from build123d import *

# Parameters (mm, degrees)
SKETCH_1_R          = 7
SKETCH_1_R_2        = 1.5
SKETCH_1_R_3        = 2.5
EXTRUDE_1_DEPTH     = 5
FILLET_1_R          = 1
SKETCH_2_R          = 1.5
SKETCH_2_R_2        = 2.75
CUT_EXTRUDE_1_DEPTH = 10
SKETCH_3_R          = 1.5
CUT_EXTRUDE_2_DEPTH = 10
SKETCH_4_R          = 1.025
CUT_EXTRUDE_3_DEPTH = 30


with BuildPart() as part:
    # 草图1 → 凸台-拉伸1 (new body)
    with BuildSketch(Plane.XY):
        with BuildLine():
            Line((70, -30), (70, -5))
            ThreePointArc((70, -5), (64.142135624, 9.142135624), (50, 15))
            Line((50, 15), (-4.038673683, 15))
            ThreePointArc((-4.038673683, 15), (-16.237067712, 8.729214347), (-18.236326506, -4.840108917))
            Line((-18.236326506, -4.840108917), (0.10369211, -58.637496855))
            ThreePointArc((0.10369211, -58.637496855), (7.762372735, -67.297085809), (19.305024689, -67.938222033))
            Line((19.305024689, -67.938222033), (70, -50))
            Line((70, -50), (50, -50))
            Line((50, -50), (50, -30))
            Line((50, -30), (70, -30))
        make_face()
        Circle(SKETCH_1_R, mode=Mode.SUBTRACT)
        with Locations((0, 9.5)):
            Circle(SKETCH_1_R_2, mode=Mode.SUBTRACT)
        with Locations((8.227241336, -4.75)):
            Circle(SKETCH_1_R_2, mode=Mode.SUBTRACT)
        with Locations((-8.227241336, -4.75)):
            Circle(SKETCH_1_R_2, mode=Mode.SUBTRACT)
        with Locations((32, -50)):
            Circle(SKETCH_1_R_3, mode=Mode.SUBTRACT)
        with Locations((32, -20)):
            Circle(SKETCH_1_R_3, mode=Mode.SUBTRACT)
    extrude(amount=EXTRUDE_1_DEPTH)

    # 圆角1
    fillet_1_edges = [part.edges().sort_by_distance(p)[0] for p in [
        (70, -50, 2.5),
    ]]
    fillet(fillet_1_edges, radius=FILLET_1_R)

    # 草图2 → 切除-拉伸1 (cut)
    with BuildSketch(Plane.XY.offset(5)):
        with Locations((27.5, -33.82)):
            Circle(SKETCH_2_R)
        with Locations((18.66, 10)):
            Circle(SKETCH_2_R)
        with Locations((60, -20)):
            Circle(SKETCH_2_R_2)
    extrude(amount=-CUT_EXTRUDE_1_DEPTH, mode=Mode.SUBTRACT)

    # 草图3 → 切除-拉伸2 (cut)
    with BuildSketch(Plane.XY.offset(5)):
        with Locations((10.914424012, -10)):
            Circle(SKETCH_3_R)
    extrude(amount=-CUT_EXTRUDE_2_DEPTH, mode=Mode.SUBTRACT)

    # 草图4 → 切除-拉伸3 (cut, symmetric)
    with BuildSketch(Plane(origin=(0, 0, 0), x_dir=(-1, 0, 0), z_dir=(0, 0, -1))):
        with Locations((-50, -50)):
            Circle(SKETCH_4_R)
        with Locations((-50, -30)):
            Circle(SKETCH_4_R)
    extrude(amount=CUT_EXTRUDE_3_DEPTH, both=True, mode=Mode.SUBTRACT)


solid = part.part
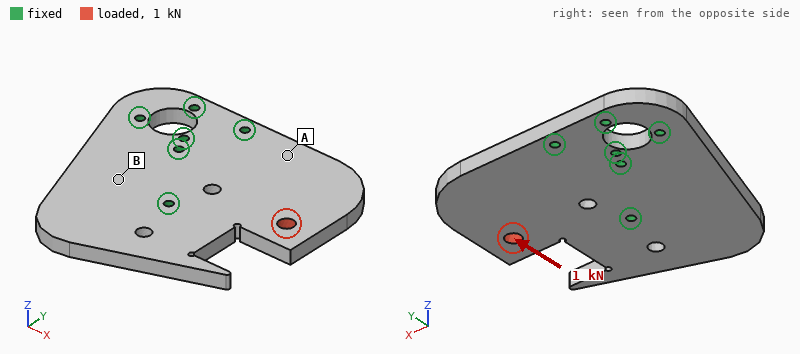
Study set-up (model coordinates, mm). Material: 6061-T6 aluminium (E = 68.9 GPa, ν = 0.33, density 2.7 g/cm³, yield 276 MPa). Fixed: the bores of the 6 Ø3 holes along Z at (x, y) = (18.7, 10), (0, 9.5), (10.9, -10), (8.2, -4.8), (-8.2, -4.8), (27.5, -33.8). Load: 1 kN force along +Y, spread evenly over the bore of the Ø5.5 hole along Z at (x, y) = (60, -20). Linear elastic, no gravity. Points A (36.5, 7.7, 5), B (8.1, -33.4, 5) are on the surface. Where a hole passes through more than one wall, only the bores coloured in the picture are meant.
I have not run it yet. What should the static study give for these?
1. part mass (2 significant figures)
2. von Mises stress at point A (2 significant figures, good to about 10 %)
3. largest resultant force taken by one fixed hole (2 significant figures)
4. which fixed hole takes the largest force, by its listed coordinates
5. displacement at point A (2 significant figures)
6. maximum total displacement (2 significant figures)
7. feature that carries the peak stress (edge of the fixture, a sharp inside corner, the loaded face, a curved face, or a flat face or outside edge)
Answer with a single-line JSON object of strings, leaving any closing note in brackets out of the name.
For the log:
{"part mass": "73 g", "von Mises stress at point A": "7.3 MPa", "largest resultant force taken by one fixed hole": "1.1 kN", "which fixed hole takes the largest force, by its listed coordinates": "(27.5, -33.8)", "displacement at point A": "4.0 µm", "maximum total displacement": "14 µm", "feature that carries the peak stress": "a curved face"}
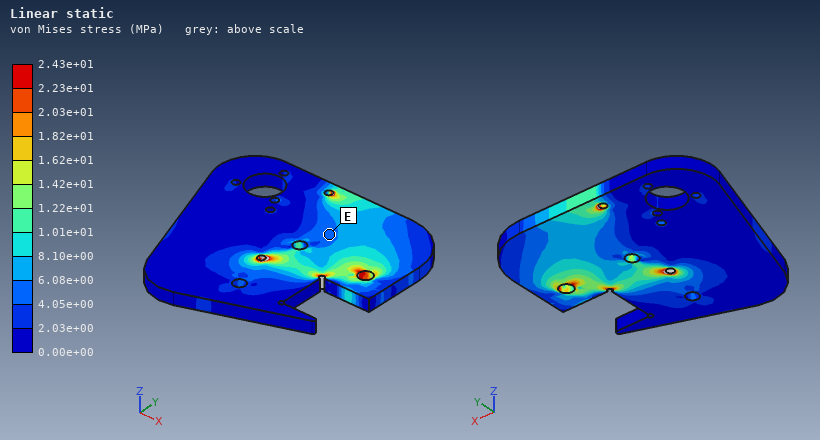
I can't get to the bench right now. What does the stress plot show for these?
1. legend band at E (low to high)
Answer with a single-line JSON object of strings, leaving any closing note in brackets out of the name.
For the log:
{"legend band at E": "4.05e+00 to 6.08e+00 MPa"}
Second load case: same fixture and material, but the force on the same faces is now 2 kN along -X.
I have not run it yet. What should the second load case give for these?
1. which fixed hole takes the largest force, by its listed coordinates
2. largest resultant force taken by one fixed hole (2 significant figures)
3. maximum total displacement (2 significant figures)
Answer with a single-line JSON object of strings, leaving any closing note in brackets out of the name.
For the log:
{"which fixed hole takes the largest force, by its listed coordinates": "(27.5, -33.8)", "largest resultant force taken by one fixed hole": "1.0 kN", "maximum total displacement": "12 µm"}
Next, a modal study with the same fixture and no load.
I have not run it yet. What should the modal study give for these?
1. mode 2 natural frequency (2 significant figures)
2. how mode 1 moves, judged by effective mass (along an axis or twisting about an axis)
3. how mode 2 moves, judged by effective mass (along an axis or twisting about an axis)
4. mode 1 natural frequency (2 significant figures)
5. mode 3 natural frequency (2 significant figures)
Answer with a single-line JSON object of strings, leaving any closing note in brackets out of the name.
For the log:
{"mode 2 natural frequency": "3100 Hz", "how mode 1 moves, judged by effective mass": "along Z", "how mode 2 moves, judged by effective mass": "along Z", "mode 1 natural frequency": "1900 Hz", "mode 3 natural frequency": "4000 Hz"}
